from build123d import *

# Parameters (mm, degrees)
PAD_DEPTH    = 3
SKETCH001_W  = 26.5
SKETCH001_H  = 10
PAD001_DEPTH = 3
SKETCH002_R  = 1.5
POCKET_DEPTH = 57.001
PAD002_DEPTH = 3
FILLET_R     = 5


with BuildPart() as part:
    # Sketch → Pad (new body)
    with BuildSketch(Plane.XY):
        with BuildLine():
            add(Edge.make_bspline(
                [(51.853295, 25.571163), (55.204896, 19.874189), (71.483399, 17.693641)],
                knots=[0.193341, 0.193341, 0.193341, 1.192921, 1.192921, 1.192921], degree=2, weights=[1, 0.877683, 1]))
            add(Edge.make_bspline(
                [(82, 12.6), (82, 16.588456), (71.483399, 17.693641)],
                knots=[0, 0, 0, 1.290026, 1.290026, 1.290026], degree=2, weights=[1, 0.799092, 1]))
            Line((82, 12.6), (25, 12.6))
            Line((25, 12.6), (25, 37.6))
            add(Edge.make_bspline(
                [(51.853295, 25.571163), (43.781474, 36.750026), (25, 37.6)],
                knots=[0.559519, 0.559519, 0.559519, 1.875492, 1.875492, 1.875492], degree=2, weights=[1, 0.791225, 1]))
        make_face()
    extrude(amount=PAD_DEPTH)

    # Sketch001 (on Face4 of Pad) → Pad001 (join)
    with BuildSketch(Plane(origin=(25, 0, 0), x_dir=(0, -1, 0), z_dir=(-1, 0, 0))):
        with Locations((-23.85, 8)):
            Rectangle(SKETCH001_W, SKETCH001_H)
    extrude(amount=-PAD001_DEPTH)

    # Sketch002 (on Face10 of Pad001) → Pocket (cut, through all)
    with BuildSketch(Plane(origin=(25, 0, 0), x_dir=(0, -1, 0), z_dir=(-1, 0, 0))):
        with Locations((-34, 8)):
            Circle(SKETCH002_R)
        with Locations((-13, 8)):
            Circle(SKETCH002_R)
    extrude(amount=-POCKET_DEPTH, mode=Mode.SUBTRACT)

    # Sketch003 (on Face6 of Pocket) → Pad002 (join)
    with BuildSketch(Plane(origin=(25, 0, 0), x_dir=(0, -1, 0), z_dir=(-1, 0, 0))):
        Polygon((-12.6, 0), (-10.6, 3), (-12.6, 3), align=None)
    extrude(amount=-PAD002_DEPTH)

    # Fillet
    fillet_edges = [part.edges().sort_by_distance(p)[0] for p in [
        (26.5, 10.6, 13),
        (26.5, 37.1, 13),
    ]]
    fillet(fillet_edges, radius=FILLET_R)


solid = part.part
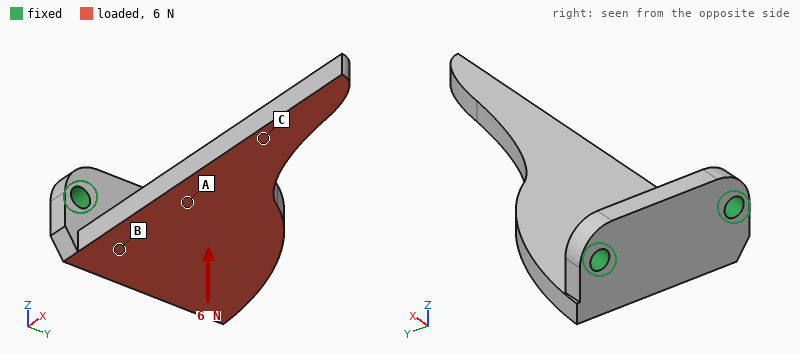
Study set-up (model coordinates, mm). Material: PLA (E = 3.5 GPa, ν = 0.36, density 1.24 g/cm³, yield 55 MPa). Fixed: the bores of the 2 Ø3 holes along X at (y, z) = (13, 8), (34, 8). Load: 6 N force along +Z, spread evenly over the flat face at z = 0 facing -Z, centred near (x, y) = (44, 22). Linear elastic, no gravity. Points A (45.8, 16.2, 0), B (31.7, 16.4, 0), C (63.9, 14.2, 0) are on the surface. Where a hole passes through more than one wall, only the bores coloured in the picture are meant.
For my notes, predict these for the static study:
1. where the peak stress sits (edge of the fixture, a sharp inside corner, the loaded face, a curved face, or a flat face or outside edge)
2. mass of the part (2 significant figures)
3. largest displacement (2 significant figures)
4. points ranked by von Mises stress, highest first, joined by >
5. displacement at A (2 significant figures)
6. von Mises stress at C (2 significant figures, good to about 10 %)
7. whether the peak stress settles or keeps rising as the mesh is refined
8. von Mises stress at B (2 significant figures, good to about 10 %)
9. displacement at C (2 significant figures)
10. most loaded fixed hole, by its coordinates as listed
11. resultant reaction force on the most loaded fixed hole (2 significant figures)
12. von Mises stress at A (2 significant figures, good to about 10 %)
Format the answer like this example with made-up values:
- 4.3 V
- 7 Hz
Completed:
- edge of the fixture
- 3.7 g
- 0.58 mm
- B > A > C
- 0.14 mm
- 0.51 MPa
- keeps rising
- 2.3 MPa
- 0.34 mm
- (13, 8)
- 3.8 N
- 1.2 MPa
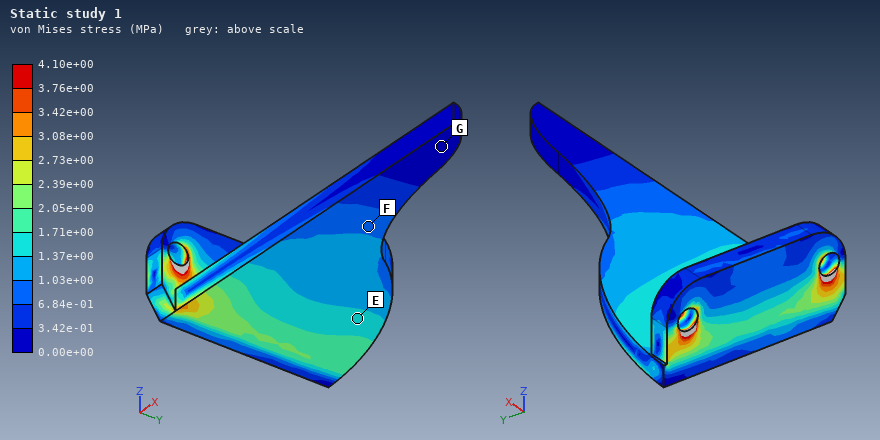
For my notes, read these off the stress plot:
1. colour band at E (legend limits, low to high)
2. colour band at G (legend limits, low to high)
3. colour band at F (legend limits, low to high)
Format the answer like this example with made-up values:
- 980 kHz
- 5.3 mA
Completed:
- 1.37e+00 to 1.71e+00 MPa
- 0.00e+00 to 3.42e-01 MPa
- 6.84e-01 to 1.03e+00 MPa
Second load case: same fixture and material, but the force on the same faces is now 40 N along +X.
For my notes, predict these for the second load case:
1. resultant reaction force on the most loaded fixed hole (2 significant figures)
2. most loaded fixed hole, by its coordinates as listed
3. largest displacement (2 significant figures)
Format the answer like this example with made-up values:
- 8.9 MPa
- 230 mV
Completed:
- 24 N
- (13, 8)
- 0.64 mm
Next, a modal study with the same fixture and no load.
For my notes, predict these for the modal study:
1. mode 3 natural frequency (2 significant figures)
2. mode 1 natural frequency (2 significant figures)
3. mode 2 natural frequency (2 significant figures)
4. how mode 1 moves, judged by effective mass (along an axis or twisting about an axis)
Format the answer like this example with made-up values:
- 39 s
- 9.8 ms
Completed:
- 1700 Hz
- 430 Hz
- 1600 Hz
- along Z
